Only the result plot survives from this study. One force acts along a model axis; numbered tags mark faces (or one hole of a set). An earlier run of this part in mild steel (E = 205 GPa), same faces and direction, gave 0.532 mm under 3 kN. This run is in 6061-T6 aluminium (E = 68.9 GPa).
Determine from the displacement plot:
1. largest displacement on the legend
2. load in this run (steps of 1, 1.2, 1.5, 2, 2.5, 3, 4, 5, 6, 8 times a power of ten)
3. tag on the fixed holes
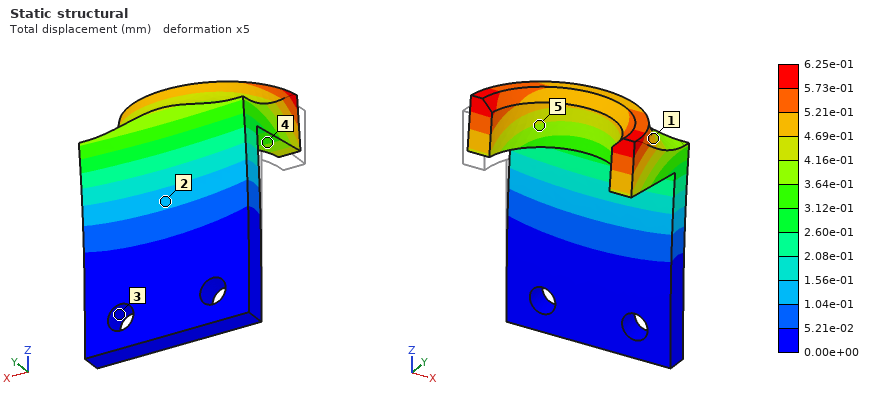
6.25e-01 mm
1.2 kN
3
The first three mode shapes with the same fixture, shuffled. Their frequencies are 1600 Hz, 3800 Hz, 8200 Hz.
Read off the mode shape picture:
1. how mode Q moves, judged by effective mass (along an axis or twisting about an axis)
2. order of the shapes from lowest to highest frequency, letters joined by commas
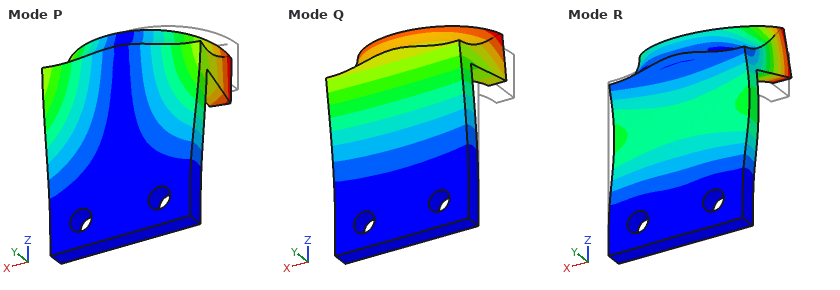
along Y
Q, P, R
